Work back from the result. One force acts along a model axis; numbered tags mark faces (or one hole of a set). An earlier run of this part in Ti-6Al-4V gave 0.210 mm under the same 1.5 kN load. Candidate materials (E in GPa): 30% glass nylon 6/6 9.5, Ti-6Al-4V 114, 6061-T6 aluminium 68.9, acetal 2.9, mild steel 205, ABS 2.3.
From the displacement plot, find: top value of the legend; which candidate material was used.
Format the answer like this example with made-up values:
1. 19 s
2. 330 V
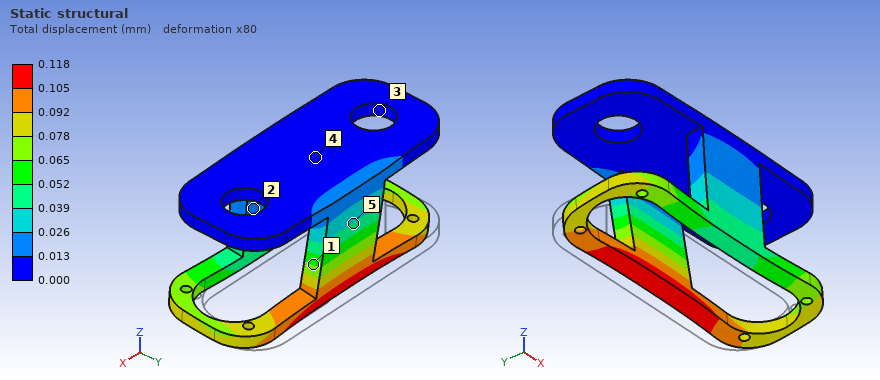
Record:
1. 0.118 mm
2. mild steel
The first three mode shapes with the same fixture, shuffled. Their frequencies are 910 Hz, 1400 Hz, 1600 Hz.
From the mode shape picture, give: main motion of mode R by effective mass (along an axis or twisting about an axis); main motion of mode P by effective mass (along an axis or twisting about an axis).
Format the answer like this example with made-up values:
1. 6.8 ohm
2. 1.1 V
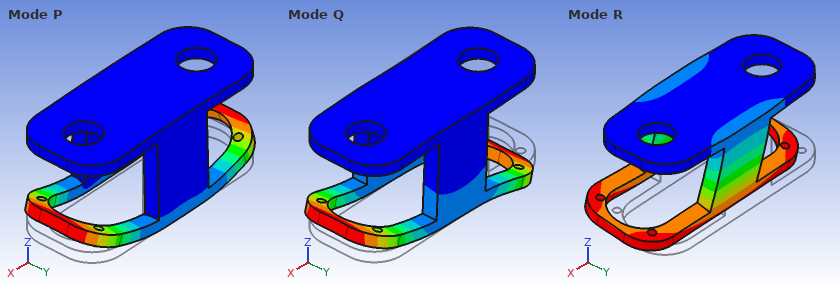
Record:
1. along Y
2. along Z
